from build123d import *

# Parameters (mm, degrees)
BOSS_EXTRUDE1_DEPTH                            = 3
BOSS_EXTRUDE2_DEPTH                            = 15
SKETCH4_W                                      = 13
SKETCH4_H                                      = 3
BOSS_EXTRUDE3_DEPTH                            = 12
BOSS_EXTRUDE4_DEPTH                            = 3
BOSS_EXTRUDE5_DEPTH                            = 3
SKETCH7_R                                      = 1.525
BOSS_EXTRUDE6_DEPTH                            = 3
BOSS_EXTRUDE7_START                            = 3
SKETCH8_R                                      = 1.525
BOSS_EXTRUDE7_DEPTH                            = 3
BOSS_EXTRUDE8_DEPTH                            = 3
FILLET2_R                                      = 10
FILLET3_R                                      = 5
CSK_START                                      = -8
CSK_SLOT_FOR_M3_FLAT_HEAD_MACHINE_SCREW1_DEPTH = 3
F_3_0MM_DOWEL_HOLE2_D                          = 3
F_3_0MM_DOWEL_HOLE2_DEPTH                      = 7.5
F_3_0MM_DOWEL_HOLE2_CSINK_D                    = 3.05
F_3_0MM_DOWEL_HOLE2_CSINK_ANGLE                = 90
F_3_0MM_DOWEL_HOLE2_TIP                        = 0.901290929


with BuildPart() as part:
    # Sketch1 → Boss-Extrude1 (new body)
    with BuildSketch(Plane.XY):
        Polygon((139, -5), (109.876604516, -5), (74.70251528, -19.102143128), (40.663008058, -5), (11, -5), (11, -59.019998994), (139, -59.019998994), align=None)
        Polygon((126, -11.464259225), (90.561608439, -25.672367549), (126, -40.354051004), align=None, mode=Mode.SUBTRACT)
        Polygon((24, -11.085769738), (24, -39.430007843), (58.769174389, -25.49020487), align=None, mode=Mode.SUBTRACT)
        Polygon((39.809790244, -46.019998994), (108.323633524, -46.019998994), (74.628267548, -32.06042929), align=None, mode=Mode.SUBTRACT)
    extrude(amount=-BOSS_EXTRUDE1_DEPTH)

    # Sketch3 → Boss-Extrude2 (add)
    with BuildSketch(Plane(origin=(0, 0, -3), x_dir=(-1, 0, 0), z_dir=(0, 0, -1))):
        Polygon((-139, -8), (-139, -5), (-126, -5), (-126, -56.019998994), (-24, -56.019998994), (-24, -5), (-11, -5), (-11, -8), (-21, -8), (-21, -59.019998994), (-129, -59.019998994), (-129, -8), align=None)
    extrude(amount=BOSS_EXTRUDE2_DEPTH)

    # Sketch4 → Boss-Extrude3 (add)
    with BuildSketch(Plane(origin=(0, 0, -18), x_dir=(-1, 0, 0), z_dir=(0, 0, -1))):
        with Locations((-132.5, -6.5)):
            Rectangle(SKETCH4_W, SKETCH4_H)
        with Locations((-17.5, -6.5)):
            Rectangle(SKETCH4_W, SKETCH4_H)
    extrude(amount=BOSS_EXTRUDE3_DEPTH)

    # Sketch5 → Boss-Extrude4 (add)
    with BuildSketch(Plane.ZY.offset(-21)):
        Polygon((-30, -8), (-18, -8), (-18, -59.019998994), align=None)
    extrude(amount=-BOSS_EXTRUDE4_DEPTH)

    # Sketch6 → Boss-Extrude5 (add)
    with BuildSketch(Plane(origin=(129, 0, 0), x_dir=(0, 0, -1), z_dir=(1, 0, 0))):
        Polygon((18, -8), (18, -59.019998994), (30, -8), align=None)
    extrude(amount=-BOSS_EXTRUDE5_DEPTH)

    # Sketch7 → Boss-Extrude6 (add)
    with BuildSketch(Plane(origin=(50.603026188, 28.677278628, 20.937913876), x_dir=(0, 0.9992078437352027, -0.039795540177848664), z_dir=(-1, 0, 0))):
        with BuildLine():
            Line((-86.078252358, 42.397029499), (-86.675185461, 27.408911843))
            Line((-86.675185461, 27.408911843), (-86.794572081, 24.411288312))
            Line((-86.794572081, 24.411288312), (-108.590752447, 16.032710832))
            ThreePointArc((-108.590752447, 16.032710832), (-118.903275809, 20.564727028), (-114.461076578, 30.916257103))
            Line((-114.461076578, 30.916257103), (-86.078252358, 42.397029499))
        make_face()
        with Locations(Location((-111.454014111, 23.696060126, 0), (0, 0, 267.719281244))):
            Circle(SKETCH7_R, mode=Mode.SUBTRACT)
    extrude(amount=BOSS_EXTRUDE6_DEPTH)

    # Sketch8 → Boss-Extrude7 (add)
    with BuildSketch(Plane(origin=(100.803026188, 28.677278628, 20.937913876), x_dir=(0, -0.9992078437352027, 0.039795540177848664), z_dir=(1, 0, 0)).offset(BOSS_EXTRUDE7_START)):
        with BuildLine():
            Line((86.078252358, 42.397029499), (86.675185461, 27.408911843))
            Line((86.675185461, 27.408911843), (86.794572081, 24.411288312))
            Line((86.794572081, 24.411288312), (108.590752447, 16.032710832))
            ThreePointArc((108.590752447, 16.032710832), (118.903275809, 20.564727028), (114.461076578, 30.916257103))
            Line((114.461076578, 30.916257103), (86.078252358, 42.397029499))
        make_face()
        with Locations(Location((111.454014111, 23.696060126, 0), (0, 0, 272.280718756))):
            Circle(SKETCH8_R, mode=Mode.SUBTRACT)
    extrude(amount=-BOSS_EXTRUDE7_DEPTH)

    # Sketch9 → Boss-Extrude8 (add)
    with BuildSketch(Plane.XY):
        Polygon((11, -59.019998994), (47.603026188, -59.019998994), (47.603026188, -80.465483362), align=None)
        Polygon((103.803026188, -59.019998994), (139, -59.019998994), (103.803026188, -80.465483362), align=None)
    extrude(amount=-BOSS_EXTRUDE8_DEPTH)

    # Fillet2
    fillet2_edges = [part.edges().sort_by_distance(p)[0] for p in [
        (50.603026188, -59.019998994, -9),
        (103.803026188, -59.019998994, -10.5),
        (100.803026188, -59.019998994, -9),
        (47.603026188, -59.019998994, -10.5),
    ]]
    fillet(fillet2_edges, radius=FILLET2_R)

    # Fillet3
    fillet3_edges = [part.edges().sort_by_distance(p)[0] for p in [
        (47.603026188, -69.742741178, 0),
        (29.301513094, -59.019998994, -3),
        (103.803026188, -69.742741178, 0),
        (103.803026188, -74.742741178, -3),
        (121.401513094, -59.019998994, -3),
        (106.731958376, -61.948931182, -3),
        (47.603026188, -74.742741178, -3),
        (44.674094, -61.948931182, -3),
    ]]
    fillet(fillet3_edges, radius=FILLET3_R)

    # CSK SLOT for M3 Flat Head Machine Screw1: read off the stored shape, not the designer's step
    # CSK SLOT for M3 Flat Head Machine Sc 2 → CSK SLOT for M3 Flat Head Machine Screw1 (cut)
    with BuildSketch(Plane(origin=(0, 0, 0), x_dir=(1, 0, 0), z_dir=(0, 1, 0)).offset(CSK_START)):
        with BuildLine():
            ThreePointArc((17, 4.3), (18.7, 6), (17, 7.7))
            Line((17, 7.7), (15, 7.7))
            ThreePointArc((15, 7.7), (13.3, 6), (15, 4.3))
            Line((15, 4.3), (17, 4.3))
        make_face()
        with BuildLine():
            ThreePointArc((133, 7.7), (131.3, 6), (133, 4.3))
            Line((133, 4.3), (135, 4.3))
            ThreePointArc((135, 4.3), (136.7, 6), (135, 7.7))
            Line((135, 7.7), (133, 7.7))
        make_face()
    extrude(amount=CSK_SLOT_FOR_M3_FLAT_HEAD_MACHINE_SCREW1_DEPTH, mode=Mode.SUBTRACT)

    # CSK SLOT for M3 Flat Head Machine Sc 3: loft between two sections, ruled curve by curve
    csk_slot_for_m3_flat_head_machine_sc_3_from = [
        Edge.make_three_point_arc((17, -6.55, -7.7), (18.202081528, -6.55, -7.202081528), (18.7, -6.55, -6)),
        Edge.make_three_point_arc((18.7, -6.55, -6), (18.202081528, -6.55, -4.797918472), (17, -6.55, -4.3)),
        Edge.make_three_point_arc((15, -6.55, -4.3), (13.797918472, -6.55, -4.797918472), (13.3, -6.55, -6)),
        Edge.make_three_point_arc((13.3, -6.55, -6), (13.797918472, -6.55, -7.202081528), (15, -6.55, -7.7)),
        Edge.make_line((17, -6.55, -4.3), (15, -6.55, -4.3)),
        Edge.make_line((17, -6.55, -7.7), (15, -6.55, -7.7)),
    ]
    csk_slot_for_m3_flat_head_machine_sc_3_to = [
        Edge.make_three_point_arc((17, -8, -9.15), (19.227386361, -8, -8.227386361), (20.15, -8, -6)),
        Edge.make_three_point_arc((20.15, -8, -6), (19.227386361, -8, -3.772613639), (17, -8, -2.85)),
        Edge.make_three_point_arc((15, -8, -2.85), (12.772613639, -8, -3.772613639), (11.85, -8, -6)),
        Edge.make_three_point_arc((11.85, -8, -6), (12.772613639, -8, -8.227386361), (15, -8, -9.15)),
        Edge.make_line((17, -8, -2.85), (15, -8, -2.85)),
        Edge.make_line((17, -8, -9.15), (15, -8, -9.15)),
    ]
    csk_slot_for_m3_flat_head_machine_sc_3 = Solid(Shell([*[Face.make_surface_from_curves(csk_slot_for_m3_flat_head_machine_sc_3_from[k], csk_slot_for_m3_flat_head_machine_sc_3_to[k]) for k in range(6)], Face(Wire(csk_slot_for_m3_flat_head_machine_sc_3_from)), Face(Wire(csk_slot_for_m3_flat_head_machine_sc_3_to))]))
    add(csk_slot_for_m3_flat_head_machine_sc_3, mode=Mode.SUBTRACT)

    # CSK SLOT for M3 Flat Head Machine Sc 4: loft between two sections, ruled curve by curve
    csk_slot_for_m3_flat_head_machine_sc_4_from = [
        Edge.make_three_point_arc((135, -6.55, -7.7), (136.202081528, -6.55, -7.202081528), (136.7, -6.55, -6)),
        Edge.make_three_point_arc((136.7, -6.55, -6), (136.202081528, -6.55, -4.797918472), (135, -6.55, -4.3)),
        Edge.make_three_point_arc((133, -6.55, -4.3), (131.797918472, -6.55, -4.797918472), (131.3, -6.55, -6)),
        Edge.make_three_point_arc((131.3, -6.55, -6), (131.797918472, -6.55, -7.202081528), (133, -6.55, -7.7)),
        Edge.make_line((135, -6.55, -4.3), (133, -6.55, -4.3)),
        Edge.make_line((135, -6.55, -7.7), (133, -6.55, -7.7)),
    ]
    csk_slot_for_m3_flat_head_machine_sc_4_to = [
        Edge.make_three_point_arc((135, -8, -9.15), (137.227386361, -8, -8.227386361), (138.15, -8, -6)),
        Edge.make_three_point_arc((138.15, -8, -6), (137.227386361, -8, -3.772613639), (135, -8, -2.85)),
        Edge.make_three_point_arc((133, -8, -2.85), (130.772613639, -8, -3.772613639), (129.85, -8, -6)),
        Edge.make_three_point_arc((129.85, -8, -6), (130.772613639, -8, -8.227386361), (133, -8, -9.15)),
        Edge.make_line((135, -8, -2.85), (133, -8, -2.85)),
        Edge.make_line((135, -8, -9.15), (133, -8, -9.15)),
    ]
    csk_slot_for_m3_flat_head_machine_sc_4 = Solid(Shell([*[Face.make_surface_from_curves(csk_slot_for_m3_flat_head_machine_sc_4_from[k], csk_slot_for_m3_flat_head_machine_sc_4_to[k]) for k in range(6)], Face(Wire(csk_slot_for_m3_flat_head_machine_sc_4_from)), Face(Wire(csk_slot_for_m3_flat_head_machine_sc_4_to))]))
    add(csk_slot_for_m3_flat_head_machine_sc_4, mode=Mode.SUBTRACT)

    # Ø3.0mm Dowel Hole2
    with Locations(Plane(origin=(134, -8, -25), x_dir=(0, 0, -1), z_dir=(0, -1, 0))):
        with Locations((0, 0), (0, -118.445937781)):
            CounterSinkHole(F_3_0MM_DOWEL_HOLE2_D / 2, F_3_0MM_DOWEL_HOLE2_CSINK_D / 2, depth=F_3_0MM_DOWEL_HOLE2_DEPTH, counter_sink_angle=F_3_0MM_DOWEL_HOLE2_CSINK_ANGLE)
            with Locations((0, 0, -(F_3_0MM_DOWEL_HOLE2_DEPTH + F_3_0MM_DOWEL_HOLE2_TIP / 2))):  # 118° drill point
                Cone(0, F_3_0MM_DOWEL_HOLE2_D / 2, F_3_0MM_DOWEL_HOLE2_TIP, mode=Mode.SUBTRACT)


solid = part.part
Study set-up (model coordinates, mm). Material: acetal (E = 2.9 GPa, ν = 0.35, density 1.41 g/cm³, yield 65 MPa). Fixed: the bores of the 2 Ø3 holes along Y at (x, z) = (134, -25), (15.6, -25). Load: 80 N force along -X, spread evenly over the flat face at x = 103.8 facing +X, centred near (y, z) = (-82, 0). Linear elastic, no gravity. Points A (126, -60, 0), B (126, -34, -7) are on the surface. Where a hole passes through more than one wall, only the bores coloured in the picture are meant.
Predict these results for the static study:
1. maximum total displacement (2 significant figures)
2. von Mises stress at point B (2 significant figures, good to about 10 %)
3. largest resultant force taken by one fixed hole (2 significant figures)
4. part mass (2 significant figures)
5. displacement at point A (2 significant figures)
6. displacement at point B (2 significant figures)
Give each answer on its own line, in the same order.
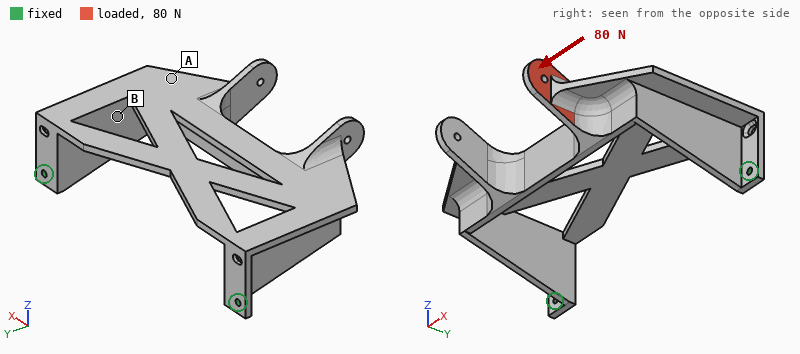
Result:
1.7 mm
3.8 MPa
68 N
50 g
1.3 mm
0.75 mm
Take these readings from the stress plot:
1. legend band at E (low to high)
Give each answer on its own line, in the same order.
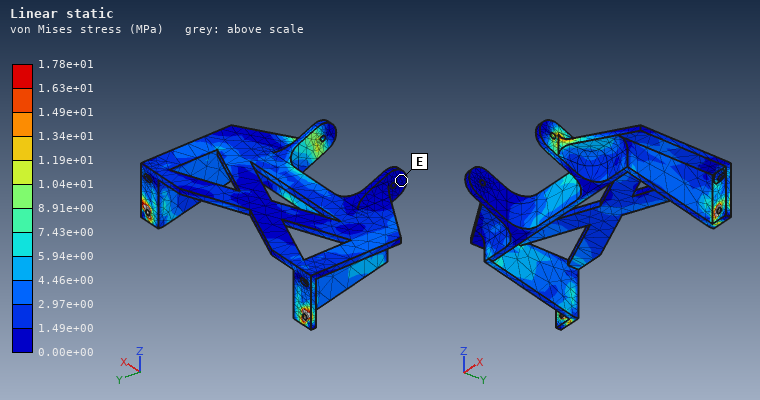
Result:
0.00e+00 to 1.49e+00 MPa
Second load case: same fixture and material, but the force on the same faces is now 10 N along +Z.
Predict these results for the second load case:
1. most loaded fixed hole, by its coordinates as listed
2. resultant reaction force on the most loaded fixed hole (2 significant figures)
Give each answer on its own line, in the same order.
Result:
(134, -25)
7.2 N
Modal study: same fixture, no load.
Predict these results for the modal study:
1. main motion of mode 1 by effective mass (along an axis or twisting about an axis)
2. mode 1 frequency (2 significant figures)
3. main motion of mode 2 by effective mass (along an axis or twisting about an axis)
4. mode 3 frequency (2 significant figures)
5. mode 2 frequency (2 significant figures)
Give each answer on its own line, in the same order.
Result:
along Z
110 Hz
along X
420 Hz
200 Hz
